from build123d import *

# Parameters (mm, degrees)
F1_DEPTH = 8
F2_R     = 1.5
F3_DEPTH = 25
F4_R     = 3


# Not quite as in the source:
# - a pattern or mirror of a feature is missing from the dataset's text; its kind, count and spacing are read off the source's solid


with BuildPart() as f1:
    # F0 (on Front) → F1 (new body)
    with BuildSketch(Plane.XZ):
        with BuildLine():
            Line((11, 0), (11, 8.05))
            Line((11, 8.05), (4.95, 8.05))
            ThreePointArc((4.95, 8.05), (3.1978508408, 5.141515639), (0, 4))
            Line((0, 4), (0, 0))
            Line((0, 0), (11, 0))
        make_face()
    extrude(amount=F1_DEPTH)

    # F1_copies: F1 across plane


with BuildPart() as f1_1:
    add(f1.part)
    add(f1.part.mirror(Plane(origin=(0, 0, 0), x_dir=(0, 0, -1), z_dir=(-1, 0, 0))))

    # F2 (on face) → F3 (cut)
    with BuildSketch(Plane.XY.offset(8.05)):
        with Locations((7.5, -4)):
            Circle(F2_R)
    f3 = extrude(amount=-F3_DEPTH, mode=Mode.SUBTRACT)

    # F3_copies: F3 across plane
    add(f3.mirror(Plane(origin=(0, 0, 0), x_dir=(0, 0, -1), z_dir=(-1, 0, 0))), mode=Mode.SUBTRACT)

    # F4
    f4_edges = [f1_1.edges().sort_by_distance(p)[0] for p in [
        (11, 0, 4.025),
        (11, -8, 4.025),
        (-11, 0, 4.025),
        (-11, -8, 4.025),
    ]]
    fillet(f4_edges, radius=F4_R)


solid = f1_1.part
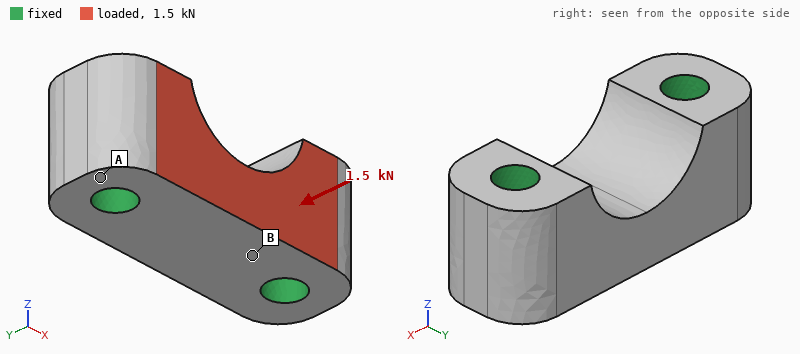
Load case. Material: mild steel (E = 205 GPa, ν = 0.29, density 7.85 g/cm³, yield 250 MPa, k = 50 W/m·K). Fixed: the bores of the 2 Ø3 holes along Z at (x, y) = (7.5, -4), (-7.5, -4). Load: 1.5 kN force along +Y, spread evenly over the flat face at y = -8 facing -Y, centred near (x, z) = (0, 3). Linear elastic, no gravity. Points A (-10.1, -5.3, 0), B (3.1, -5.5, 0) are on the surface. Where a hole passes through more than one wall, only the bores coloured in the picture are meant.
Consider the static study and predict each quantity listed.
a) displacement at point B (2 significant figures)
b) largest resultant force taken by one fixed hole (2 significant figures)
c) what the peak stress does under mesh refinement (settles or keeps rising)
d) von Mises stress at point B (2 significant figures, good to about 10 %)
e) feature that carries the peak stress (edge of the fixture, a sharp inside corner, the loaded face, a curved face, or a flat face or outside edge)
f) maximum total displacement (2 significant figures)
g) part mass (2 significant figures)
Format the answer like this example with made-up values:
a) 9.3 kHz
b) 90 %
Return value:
a) 0.78 µm
b) 760 N
c) keeps rising
d) 18 MPa
e) edge of the fixture
f) 1.2 µm
g) 7.9 g
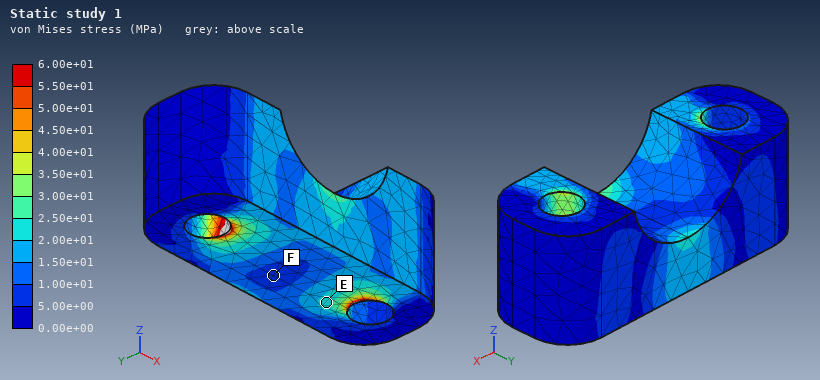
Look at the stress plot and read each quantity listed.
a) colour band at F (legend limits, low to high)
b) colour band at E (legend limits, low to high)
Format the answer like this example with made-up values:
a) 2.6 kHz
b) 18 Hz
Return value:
a) 5.00e+00 to 1.00e+01 MPa
b) 2.00e+01 to 2.50e+01 MPa
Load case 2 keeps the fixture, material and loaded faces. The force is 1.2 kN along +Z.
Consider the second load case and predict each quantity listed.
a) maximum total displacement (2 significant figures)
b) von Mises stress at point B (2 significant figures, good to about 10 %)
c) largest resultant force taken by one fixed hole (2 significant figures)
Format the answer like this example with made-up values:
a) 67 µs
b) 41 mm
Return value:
a) 2.2 µm
b) 24 MPa
c) 600 N
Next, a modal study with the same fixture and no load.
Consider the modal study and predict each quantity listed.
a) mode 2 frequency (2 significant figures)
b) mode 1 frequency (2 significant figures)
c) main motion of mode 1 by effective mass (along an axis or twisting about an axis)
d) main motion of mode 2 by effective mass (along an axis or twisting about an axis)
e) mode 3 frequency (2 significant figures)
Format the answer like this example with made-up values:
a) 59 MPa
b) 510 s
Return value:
a) 110 kHz
b) 94 kHz
c) along Y
d) along Z
e) 130 kHz
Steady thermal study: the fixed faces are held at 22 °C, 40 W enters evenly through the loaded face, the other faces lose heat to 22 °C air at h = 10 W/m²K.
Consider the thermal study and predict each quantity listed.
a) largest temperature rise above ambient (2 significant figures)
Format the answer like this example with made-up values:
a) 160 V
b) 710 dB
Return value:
a) 43 K
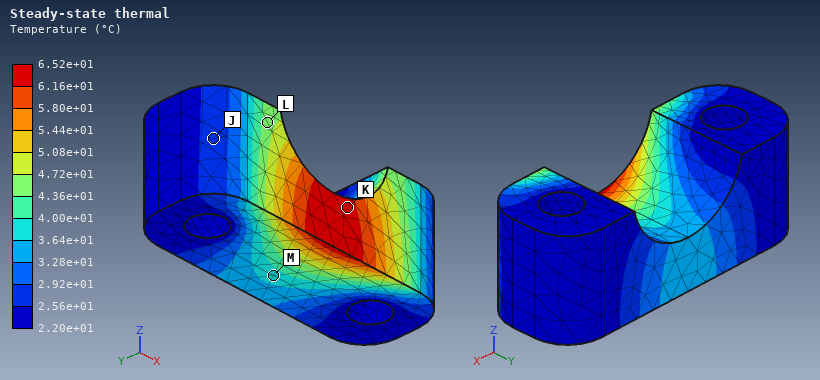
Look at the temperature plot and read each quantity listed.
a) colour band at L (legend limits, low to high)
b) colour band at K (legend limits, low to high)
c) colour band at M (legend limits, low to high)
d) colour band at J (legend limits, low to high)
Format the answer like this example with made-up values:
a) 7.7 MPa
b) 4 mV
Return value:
a) 4.36e+01 to 4.72e+01 °C
b) 6.16e+01 to 6.52e+01 °C
c) 3.64e+01 to 4.00e+01 °C
d) 2.56e+01 to 2.92e+01 °C
